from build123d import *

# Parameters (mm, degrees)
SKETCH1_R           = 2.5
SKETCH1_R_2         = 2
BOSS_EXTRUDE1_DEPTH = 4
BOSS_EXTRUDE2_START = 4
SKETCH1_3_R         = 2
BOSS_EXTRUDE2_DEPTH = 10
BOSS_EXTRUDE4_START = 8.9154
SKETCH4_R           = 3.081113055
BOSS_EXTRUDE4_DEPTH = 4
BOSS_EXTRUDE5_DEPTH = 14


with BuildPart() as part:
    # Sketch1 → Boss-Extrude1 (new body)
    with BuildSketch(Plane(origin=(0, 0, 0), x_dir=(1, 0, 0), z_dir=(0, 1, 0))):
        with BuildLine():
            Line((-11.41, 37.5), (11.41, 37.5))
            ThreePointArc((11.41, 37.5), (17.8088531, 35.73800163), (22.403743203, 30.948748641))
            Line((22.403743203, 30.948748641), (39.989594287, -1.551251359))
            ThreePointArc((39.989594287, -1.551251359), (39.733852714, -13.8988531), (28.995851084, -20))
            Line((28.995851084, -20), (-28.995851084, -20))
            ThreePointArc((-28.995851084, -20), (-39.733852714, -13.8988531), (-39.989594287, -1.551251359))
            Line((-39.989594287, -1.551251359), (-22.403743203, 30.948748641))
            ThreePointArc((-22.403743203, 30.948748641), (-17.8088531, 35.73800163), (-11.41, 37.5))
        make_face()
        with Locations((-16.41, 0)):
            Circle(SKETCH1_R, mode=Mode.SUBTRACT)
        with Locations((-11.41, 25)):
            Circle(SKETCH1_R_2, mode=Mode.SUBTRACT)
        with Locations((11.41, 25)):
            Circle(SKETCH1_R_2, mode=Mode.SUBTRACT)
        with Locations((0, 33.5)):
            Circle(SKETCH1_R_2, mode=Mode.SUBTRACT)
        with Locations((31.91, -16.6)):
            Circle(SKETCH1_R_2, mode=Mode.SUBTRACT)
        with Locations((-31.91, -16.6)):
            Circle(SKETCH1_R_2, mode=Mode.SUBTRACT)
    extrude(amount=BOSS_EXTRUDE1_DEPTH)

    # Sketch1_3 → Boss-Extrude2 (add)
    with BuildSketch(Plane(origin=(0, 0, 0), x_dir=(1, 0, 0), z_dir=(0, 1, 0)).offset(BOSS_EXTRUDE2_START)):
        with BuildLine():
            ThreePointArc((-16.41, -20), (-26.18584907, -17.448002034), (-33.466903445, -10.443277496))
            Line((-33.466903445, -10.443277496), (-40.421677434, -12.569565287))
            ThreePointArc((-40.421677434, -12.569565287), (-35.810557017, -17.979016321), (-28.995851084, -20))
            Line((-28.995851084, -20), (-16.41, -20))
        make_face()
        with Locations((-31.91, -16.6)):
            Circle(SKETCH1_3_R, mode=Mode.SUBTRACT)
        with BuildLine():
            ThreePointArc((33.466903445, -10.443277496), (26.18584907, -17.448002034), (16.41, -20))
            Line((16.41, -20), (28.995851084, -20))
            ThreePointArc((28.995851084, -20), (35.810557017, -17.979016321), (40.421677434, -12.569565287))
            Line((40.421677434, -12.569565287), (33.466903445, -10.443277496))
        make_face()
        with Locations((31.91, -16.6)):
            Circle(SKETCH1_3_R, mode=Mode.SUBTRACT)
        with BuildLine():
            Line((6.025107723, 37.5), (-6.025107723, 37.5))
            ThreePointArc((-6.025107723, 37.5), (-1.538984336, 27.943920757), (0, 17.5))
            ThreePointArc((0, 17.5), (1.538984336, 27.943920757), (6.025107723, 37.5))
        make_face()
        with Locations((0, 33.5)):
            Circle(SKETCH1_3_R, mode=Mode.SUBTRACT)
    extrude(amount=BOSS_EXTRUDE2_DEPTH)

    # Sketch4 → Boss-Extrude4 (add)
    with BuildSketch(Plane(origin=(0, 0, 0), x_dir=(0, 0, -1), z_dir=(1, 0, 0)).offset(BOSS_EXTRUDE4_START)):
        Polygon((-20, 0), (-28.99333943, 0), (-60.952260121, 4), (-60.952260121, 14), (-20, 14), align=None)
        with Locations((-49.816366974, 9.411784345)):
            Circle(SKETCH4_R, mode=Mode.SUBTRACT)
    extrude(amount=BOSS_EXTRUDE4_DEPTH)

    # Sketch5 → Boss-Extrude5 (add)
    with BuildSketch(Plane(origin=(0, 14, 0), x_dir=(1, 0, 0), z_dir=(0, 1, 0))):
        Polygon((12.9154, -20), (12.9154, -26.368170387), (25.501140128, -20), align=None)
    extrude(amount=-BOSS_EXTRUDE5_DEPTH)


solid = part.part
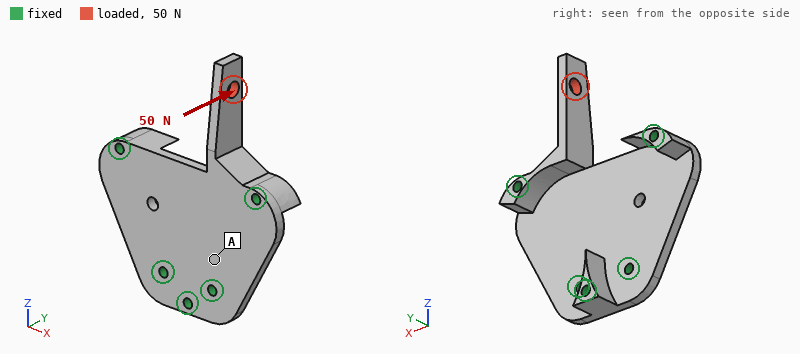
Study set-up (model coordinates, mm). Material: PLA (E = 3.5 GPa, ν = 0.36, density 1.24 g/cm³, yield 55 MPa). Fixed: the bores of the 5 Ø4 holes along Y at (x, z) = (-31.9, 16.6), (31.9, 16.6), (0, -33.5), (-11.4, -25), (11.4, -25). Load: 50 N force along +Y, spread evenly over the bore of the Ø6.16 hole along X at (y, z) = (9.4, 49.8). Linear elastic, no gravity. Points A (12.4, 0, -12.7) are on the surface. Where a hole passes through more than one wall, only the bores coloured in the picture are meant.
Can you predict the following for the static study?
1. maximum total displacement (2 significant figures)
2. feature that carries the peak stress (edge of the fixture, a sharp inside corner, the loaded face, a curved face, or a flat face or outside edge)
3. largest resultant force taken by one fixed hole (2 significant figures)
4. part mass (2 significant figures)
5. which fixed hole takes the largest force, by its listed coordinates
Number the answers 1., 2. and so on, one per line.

1. 1.4 mm
2. a curved face
3. 78 N
4. 24 g
5. (31.9, 16.6)
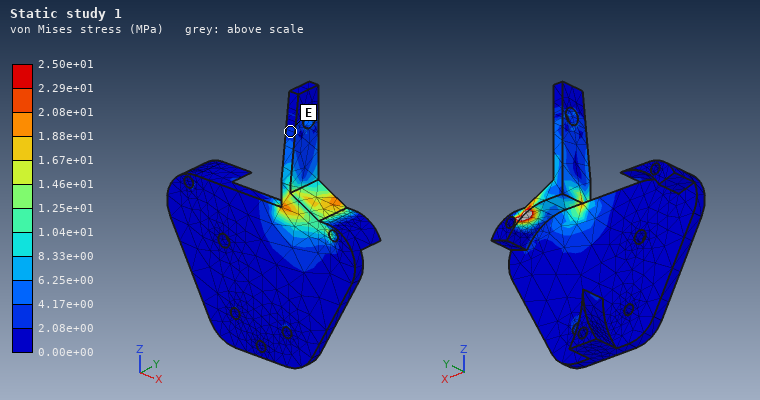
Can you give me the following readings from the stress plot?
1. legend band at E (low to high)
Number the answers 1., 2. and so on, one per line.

1. 2.08e+00 to 4.17e+00 MPa
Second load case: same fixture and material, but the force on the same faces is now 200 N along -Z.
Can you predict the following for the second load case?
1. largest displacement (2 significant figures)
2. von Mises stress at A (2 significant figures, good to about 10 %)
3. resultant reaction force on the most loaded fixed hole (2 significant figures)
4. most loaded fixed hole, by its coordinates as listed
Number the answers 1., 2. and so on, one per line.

1. 1.3 mm
2. 1.7 MPa
3. 81 N
4. (31.9, 16.6)
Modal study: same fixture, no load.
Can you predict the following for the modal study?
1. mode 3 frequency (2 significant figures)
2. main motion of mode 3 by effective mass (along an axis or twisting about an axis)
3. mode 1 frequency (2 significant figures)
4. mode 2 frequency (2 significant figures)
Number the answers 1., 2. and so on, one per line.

1. 2400 Hz
2. along Y
3. 830 Hz
4. 1000 Hz
